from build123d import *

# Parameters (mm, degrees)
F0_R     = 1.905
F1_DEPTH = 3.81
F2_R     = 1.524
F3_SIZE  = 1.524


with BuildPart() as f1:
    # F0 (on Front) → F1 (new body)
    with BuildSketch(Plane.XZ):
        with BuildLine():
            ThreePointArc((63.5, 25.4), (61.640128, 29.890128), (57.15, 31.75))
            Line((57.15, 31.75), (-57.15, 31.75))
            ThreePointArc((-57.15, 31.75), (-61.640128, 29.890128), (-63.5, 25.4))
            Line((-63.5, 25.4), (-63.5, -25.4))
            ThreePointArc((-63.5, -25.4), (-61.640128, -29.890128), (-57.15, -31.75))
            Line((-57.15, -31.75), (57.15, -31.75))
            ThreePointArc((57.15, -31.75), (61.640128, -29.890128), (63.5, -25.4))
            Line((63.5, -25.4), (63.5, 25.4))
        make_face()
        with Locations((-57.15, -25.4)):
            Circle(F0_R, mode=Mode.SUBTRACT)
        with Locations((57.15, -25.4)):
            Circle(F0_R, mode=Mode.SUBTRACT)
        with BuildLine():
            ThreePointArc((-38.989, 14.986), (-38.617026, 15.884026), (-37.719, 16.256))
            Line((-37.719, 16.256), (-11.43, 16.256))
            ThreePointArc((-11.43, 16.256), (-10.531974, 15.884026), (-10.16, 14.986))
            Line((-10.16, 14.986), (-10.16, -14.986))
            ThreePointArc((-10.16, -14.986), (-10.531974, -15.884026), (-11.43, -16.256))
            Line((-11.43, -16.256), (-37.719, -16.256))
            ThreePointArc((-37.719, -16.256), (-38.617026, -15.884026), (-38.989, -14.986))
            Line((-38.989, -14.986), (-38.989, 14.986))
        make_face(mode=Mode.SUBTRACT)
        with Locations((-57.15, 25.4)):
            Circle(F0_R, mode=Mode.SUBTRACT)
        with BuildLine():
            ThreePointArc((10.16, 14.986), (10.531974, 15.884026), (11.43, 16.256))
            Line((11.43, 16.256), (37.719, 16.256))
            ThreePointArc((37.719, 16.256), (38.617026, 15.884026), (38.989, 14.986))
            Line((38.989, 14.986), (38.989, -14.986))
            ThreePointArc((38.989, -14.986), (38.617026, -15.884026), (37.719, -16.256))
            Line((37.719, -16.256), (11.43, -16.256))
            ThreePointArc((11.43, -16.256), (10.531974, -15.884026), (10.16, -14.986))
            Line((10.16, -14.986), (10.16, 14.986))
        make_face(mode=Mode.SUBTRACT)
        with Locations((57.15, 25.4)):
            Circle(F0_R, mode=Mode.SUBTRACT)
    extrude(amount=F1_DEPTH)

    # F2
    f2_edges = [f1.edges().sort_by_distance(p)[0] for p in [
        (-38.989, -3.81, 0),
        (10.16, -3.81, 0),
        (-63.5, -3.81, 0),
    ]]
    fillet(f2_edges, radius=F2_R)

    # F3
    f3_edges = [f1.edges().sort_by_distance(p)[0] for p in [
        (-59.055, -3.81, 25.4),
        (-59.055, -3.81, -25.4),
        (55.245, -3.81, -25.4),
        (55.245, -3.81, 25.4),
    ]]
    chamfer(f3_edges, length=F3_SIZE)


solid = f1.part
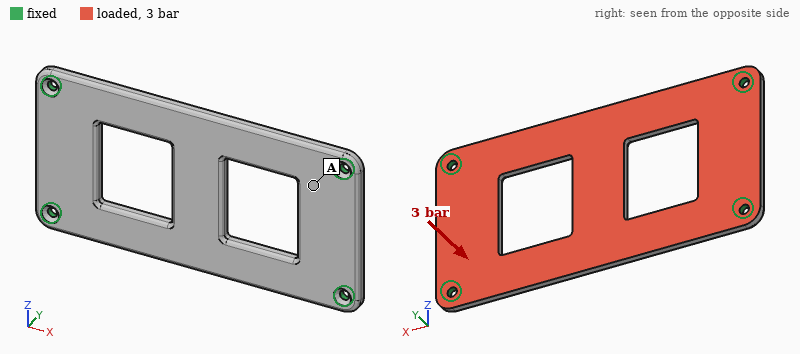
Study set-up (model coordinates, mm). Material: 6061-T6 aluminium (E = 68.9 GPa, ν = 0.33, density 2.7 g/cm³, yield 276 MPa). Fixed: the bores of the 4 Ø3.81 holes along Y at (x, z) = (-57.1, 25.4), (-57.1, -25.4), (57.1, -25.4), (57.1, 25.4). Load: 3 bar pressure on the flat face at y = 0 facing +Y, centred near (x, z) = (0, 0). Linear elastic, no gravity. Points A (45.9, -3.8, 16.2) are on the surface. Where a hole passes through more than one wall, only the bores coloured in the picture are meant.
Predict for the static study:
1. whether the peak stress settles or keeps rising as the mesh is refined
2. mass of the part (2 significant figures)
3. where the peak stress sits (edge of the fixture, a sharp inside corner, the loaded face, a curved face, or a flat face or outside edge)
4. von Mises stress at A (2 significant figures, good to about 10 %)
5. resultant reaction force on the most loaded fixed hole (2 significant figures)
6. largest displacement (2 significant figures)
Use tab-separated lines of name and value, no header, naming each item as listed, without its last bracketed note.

whether the peak stress settles or keeps rising as the mesh is refined	keeps rising
mass of the part	62 g
where the peak stress sits	edge of the fixture
von Mises stress at A	47 MPa
resultant reaction force on the most loaded fixed hole	520 N
largest displacement	0.60 mm
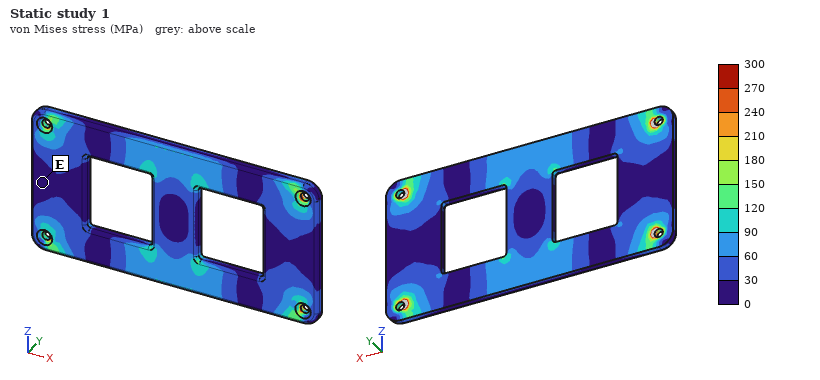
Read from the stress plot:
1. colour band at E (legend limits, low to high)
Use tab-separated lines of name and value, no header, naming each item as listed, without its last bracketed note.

colour band at E	0 to 30 MPa
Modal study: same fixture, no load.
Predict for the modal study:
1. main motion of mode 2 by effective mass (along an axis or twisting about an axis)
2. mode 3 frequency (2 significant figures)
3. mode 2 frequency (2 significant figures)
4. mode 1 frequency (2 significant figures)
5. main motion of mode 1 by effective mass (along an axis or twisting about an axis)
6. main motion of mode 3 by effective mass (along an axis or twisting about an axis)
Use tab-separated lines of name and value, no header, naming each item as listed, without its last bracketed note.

main motion of mode 2 by effective mass	twisting about X
mode 3 frequency	3600 Hz
mode 2 frequency	1900 Hz
mode 1 frequency	1300 Hz
main motion of mode 1 by effective mass	along Y
main motion of mode 3 by effective mass	twisting about Z
